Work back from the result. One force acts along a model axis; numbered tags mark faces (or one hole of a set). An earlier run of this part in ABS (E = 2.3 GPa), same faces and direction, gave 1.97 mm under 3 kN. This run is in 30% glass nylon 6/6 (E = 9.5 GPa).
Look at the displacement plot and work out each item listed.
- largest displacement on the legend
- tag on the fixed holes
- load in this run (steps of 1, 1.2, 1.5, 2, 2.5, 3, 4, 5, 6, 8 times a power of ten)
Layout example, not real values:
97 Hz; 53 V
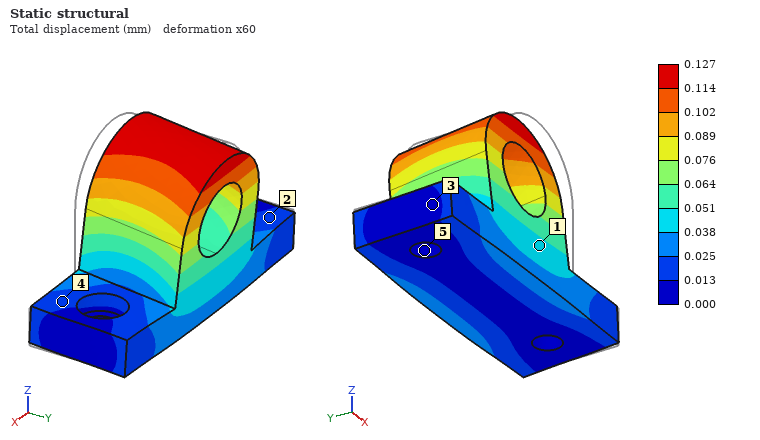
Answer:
0.127 mm; 5; 800 N
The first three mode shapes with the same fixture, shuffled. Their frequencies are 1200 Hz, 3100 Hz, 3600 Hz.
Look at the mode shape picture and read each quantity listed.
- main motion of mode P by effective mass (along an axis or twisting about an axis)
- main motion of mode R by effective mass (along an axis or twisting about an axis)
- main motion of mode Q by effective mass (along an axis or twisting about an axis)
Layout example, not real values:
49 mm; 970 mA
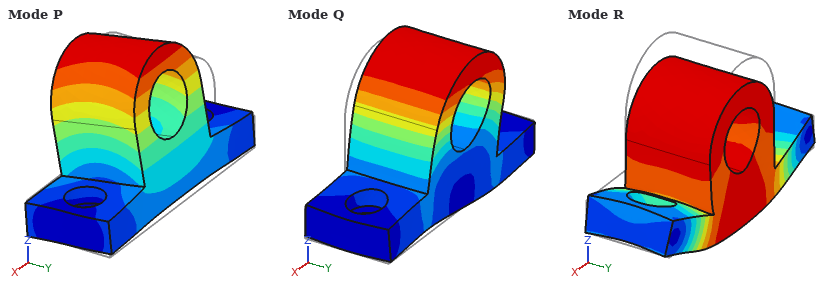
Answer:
along Y; along Z; along X
